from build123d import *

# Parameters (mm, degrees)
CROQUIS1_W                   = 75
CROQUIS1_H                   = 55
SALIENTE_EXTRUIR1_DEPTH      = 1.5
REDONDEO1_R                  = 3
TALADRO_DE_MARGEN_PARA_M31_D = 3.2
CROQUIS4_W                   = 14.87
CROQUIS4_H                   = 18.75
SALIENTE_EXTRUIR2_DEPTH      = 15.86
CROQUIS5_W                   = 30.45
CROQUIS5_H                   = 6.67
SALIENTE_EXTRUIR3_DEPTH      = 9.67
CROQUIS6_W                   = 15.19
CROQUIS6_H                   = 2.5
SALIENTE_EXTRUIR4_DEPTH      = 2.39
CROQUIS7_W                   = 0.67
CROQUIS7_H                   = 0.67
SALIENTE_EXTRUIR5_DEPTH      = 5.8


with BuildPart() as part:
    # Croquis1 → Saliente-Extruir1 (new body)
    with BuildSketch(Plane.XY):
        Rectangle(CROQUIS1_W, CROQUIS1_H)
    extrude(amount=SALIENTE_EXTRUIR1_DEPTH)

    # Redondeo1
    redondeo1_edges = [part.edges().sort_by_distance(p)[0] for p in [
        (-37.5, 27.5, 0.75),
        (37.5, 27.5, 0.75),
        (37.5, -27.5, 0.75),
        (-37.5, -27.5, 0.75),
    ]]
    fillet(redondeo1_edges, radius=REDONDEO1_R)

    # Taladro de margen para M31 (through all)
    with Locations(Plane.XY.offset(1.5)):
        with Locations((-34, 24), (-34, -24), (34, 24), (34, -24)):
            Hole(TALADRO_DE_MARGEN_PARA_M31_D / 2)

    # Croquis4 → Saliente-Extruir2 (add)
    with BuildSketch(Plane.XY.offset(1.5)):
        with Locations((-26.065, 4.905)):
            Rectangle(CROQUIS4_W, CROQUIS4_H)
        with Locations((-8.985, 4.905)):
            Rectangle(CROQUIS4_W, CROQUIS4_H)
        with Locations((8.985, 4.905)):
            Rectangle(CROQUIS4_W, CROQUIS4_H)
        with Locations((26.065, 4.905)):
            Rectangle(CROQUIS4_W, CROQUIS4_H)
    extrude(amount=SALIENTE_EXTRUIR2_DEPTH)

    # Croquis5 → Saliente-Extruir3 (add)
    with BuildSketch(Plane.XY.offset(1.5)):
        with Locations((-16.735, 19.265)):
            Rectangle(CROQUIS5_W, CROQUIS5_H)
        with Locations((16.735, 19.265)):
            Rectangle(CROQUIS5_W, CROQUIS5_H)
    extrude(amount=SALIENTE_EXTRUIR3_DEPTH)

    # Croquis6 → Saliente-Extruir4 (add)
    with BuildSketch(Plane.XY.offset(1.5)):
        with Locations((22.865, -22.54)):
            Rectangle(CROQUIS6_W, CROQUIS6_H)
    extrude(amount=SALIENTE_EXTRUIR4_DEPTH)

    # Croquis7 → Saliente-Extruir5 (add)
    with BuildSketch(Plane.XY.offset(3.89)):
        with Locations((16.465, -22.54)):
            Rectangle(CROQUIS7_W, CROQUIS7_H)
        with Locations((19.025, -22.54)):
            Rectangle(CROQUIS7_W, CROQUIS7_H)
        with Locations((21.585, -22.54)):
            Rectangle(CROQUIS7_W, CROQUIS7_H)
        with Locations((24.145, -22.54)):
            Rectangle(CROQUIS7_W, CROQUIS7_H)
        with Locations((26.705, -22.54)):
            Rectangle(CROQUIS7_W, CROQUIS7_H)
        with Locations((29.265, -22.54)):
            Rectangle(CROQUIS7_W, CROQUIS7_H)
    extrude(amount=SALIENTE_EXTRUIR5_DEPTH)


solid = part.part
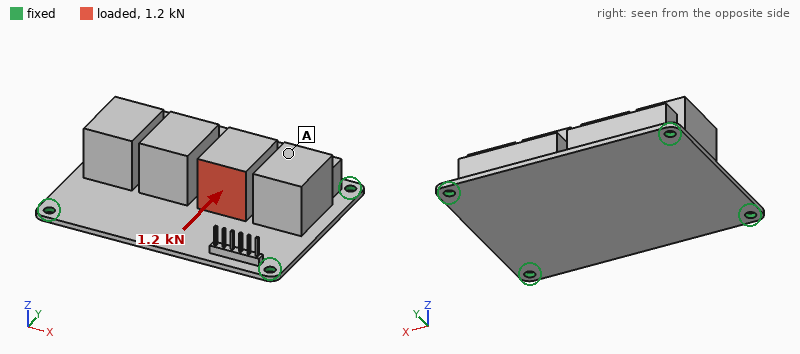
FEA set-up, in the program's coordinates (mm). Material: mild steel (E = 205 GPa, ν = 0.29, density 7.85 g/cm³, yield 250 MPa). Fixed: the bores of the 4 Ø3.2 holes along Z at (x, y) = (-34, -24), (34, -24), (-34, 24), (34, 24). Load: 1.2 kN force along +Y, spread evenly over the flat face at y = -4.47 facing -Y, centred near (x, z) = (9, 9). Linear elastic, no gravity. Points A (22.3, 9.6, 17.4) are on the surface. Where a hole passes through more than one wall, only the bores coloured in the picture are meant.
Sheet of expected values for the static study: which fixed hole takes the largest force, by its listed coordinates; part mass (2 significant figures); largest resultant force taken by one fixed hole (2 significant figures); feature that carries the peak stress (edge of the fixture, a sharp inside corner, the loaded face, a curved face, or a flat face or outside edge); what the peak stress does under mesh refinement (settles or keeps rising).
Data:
(34, 24)
220 g
510 N
edge of the fixture
keeps rising
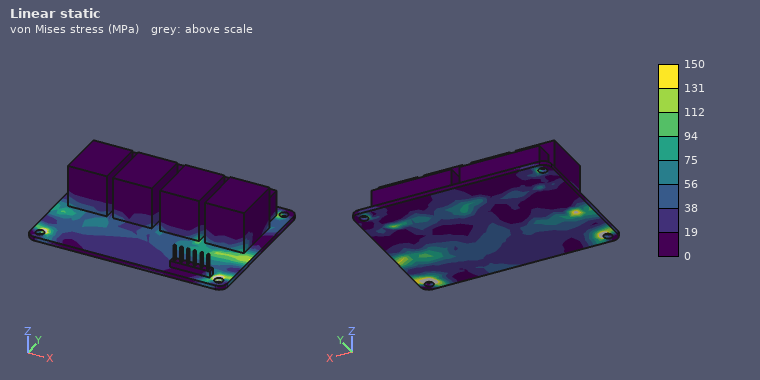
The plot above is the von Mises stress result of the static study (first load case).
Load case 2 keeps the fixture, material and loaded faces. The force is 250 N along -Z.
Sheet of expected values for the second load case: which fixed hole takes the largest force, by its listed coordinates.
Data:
(34, 24)
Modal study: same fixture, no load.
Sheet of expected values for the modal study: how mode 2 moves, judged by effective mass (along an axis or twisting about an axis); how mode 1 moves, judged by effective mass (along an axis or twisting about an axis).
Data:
along Y
along Z
